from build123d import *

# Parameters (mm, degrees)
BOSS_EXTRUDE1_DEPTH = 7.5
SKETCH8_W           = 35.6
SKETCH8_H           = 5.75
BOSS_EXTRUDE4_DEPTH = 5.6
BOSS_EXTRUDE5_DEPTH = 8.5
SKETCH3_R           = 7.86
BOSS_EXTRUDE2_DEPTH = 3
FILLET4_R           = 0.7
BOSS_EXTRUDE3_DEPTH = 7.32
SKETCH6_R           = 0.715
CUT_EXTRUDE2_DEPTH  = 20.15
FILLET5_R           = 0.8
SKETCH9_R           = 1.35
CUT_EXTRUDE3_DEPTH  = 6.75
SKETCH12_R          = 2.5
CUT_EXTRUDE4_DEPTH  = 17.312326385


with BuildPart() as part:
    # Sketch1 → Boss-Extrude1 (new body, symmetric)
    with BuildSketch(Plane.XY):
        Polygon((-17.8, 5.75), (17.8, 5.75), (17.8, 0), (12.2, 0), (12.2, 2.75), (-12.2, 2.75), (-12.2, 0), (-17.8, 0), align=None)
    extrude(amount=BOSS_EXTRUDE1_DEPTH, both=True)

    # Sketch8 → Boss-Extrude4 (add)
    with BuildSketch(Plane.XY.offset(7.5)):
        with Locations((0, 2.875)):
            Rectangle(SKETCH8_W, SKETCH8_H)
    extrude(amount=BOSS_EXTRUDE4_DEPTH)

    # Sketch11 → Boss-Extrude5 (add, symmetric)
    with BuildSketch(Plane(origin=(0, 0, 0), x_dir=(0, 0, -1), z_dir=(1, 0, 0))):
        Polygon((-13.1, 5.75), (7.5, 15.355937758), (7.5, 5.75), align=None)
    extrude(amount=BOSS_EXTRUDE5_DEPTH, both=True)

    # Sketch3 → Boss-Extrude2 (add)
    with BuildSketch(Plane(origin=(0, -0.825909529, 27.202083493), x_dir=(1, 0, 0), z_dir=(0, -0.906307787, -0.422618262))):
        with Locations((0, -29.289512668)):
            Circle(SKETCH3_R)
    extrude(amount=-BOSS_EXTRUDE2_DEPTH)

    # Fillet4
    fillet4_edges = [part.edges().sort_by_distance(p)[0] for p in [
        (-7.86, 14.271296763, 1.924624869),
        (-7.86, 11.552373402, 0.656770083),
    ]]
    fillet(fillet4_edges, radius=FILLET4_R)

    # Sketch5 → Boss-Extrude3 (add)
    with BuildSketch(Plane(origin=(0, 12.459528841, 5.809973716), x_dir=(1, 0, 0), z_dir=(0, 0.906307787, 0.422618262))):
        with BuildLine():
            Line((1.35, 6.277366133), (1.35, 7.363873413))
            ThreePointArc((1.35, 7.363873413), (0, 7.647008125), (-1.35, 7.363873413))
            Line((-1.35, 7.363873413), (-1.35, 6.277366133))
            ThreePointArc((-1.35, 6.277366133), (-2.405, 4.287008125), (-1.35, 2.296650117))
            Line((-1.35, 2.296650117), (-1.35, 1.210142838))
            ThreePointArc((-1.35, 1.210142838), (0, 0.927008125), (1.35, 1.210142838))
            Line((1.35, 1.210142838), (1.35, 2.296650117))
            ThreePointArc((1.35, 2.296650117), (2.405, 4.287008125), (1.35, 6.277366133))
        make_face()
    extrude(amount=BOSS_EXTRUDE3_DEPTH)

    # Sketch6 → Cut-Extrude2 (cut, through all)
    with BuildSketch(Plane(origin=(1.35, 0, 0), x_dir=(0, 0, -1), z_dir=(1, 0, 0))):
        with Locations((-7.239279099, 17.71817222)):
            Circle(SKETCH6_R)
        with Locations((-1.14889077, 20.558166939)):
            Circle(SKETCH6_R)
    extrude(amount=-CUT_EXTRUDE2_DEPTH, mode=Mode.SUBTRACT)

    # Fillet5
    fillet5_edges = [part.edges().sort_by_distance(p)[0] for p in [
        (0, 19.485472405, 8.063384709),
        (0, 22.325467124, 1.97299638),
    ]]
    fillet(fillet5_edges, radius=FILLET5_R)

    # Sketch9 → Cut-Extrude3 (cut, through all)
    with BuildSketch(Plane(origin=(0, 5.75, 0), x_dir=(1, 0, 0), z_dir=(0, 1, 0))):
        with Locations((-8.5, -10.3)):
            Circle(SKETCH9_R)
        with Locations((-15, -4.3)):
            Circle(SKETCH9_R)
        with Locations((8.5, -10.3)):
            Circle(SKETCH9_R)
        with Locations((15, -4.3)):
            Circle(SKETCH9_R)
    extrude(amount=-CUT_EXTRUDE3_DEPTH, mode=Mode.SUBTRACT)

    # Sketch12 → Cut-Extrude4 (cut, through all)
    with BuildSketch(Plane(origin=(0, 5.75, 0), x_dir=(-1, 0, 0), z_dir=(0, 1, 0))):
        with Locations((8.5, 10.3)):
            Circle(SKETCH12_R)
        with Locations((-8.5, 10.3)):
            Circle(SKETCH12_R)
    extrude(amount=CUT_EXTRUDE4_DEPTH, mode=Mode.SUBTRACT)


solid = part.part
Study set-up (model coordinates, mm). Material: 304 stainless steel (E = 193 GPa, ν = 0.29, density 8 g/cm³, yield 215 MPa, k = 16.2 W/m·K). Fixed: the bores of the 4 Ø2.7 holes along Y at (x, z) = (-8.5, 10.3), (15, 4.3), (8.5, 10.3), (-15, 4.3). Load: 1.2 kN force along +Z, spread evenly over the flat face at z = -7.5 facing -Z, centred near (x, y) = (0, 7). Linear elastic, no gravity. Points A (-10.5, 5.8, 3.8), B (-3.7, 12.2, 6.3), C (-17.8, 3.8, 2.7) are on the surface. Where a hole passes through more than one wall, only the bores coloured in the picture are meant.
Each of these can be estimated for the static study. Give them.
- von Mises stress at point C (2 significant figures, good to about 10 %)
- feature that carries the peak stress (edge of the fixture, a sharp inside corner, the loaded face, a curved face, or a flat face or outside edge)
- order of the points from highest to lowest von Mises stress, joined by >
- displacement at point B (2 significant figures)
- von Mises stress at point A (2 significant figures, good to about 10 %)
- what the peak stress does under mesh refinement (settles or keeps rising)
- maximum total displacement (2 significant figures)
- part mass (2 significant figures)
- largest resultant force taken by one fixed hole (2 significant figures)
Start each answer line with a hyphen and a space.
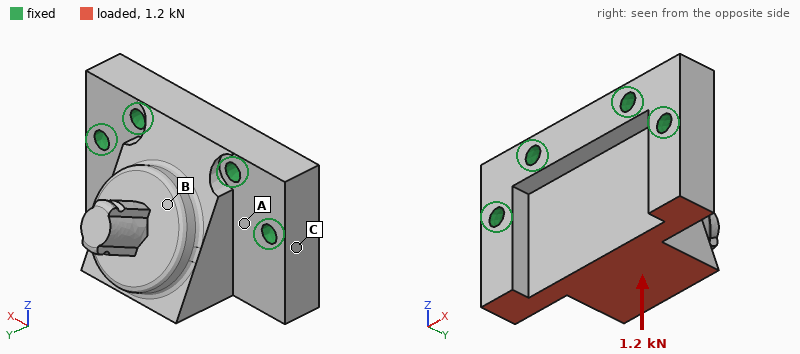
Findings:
- 10 MPa
- edge of the fixture
- A > C > B
- 2.7 µm
- 19 MPa
- keeps rising
- 5.6 µm
- 44 g
- 460 N
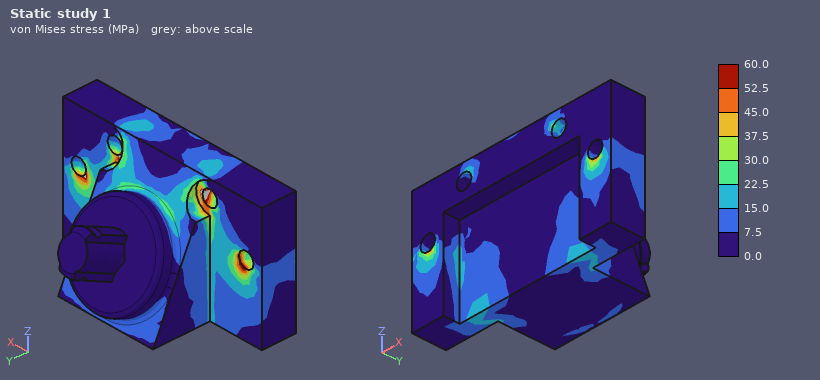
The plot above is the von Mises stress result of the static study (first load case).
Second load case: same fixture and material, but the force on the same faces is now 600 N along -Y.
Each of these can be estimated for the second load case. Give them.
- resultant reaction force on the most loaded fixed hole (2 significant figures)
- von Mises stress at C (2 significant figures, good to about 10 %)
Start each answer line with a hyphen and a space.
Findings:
- 430 N
- 17 MPa
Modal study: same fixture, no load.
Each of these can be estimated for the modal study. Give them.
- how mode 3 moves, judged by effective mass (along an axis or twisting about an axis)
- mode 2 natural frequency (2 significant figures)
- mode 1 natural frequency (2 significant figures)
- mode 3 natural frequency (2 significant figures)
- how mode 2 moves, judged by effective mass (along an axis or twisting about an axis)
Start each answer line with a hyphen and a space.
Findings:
- along X
- 25 kHz
- 11 kHz
- 35 kHz
- along X
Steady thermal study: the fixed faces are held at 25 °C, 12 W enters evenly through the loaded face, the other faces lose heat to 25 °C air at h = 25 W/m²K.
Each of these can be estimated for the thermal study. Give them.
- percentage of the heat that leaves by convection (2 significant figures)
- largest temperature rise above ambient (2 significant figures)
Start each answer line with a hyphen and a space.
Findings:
- 11 %
- 57 K
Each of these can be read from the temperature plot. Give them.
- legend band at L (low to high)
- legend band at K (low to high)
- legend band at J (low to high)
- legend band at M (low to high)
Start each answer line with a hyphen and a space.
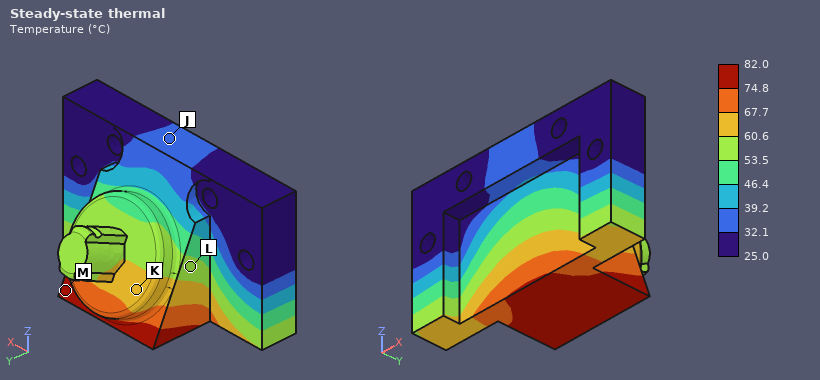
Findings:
- 53.5 to 60.6 °C
- 60.6 to 67.7 °C
- 32.1 to 39.2 °C
- 74.8 to 82.0 °C
